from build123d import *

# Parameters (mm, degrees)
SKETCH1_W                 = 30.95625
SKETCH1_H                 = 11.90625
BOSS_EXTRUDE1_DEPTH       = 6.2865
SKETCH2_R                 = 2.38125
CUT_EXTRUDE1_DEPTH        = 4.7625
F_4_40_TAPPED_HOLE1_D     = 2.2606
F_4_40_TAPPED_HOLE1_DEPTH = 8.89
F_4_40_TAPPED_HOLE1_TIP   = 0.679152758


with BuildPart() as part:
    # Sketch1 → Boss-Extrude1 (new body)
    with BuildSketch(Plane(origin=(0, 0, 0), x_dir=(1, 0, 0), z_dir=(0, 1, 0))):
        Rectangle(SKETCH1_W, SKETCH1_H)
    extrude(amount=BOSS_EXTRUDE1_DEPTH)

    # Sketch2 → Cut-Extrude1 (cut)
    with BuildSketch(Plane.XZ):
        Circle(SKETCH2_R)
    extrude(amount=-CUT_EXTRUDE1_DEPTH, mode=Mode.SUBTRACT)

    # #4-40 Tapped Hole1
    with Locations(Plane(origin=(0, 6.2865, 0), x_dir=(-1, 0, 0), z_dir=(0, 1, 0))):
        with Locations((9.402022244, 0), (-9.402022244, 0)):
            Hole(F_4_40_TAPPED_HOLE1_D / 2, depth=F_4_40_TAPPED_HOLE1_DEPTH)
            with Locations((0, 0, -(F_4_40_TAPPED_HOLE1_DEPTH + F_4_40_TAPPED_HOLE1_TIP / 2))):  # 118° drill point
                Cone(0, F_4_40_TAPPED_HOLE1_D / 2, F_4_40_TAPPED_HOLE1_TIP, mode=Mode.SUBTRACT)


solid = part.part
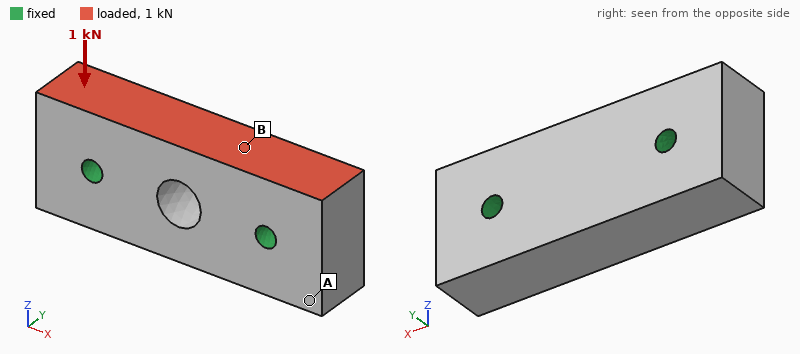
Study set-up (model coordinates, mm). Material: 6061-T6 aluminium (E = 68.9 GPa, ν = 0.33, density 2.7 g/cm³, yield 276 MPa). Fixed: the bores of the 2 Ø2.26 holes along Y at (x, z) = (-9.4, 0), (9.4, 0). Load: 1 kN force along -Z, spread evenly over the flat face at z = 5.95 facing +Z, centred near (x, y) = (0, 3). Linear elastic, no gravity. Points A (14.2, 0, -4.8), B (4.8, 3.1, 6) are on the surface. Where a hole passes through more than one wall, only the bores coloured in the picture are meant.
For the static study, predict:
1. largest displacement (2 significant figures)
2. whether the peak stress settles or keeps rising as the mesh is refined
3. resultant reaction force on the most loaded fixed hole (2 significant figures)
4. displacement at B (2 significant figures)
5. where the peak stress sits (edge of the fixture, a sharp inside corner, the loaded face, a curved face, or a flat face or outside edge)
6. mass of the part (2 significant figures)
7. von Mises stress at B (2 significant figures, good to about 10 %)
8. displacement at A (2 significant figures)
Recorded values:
1.6 µm
keeps rising
500 N
1.1 µm
edge of the fixture
5.9 g
4.5 MPa
0.29 µm
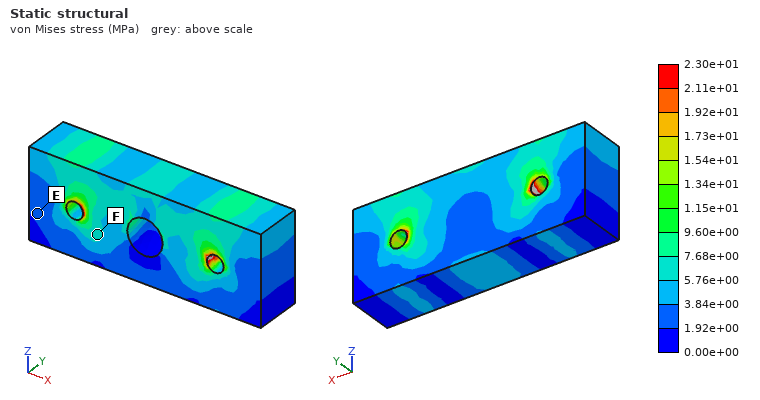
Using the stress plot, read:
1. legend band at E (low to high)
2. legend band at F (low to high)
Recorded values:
1.92e+00 to 3.84e+00 MPa
5.76e+00 to 7.68e+00 MPa
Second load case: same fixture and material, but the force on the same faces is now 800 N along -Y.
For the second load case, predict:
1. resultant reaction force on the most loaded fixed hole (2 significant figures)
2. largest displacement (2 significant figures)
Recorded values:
400 N
6.6 µm
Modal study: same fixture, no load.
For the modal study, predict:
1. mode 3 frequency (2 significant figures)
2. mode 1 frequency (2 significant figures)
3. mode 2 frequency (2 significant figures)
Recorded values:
55 kHz
52 kHz
53 kHz
